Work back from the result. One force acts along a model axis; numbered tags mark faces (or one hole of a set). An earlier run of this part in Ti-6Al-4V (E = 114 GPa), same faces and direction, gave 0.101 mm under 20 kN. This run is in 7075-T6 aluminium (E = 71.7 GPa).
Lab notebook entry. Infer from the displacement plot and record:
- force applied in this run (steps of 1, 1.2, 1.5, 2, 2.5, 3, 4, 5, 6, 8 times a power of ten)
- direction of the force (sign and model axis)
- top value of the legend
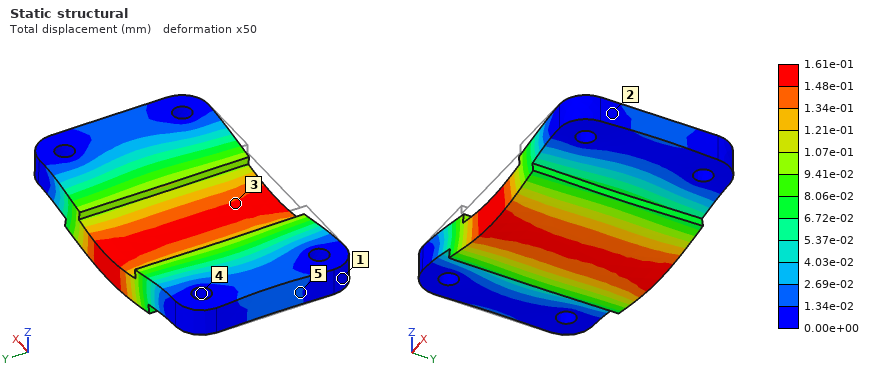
20 kN
-Z
1.61e-01 mm
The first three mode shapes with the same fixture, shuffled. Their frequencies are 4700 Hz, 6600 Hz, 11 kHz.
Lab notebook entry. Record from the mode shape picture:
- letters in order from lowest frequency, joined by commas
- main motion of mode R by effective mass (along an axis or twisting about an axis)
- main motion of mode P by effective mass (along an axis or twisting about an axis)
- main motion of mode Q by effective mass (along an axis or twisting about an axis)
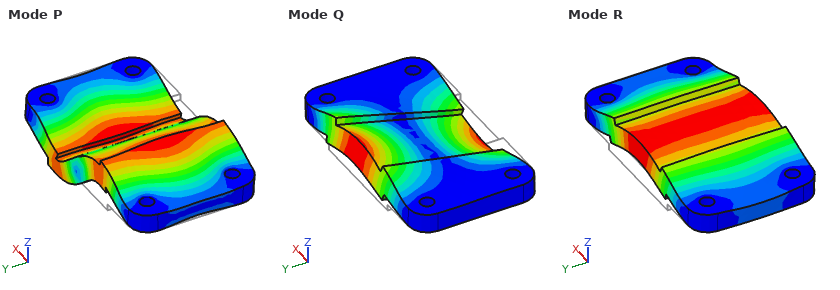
R, Q, P
along Z
twisting about Y
twisting about X
